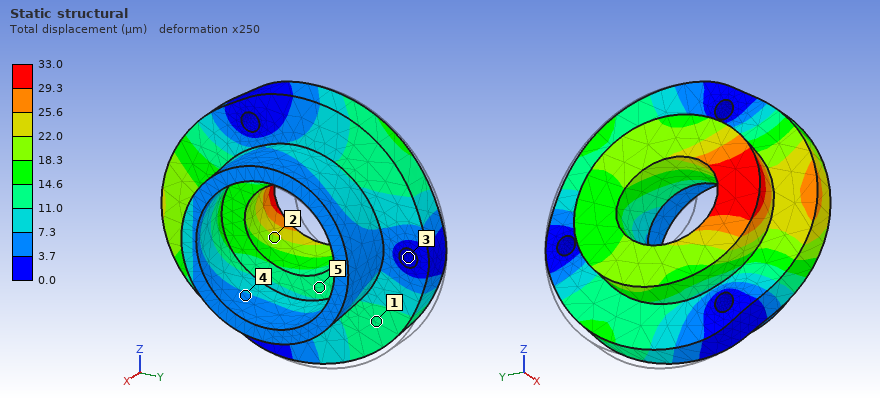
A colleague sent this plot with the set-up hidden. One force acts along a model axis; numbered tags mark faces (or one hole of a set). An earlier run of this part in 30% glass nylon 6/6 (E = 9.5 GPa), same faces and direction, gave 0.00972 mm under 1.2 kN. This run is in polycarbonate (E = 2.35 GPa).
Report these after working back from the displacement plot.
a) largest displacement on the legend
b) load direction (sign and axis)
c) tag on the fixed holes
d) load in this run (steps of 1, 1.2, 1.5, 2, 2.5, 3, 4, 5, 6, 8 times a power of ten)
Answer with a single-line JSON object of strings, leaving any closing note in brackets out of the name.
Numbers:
{"largest displacement on the legend": "33.0 µm", "load direction": "-Y", "tag on the fixed holes": "3", "load in this run": "1 kN"}
